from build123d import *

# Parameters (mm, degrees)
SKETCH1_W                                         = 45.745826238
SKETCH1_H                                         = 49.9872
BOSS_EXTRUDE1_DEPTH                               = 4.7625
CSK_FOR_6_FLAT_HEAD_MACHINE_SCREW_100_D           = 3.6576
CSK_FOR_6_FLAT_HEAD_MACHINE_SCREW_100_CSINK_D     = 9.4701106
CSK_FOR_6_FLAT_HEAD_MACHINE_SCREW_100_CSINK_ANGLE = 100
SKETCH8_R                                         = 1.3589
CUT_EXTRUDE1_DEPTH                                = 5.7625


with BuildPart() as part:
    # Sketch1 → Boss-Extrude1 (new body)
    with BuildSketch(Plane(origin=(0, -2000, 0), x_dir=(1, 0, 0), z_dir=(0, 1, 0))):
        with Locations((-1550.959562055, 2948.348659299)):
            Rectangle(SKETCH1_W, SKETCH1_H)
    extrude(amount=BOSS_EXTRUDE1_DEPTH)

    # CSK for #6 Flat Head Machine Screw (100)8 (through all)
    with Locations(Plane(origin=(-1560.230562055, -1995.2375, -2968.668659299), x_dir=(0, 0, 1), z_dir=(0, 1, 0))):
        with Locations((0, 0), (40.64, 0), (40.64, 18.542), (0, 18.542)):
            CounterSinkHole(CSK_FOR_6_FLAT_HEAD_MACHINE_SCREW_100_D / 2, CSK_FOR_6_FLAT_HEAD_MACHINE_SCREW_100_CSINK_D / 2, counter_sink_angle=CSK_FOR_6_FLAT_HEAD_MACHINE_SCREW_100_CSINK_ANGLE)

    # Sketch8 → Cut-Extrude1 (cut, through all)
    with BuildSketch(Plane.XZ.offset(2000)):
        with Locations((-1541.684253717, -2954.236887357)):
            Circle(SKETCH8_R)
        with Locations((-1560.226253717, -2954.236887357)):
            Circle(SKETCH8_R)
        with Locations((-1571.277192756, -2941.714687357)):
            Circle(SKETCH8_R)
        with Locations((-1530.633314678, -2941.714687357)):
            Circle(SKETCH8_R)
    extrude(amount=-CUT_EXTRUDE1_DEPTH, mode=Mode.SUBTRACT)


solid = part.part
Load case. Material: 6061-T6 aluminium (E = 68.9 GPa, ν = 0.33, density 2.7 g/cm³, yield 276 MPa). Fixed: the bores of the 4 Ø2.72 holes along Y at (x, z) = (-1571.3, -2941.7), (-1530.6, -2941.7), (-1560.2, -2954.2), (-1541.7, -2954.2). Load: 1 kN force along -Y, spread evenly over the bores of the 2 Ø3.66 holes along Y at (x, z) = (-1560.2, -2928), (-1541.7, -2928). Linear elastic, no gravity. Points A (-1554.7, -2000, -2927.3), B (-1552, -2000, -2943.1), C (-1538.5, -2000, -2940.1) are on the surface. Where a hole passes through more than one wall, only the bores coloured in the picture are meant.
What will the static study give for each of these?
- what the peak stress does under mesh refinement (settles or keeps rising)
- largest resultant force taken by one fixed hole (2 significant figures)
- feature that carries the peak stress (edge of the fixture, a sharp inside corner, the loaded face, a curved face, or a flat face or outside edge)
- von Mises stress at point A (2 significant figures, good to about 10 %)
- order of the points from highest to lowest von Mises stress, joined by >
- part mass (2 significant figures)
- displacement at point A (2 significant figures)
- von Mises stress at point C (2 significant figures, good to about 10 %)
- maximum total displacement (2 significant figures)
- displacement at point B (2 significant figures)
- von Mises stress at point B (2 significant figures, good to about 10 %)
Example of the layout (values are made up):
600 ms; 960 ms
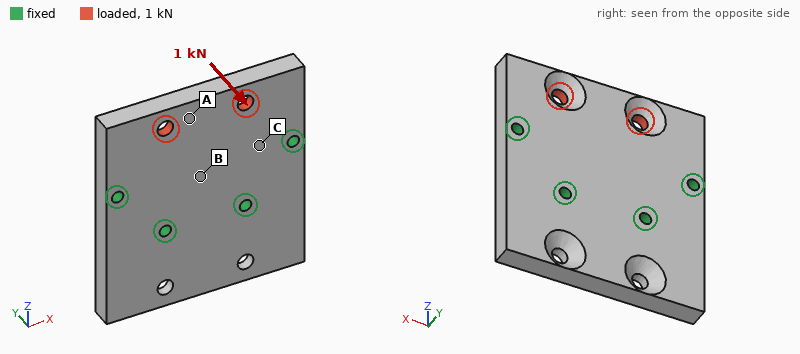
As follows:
keeps rising; 580 N; edge of the fixture; 17 MPa; C > B > A; 28 g; 0.094 mm; 58 MPa; 0.12 mm; 0.020 mm; 44 MPa
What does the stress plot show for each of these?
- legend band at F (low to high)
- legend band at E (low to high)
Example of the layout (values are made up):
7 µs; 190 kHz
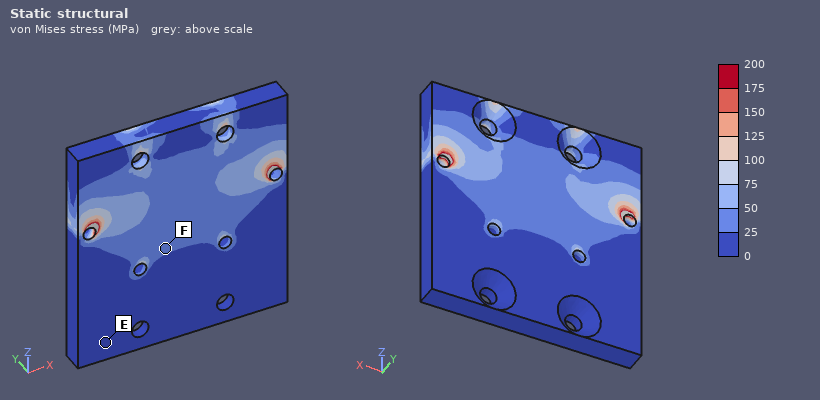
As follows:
25 to 50 MPa; 0 to 25 MPa
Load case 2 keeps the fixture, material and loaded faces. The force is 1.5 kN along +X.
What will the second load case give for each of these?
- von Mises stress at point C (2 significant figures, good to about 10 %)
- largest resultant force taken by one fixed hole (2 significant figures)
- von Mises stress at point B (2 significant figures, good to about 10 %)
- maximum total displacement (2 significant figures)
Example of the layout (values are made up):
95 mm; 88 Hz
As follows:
14 MPa; 790 N; 8.2 MPa; 8.9 µm
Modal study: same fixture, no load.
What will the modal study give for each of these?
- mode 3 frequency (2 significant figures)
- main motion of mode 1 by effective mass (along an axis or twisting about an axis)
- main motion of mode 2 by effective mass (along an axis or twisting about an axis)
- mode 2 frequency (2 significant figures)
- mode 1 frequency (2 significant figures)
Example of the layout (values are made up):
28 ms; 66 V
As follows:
11 kHz; along Y; along Y; 9300 Hz; 7800 Hz
